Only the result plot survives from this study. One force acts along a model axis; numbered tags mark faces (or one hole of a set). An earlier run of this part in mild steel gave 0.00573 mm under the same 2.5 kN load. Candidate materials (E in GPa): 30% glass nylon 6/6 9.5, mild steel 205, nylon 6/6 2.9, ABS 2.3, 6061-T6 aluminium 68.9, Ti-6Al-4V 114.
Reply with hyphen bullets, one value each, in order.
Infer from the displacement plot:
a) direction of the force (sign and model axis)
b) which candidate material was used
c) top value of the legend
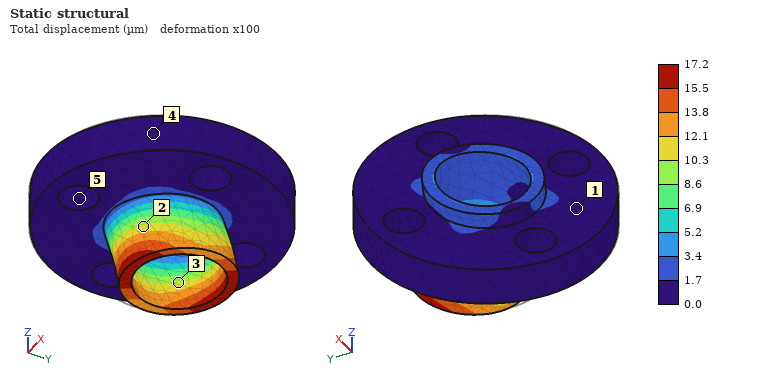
- +Y
- 6061-T6 aluminium
- 17.2 µm
